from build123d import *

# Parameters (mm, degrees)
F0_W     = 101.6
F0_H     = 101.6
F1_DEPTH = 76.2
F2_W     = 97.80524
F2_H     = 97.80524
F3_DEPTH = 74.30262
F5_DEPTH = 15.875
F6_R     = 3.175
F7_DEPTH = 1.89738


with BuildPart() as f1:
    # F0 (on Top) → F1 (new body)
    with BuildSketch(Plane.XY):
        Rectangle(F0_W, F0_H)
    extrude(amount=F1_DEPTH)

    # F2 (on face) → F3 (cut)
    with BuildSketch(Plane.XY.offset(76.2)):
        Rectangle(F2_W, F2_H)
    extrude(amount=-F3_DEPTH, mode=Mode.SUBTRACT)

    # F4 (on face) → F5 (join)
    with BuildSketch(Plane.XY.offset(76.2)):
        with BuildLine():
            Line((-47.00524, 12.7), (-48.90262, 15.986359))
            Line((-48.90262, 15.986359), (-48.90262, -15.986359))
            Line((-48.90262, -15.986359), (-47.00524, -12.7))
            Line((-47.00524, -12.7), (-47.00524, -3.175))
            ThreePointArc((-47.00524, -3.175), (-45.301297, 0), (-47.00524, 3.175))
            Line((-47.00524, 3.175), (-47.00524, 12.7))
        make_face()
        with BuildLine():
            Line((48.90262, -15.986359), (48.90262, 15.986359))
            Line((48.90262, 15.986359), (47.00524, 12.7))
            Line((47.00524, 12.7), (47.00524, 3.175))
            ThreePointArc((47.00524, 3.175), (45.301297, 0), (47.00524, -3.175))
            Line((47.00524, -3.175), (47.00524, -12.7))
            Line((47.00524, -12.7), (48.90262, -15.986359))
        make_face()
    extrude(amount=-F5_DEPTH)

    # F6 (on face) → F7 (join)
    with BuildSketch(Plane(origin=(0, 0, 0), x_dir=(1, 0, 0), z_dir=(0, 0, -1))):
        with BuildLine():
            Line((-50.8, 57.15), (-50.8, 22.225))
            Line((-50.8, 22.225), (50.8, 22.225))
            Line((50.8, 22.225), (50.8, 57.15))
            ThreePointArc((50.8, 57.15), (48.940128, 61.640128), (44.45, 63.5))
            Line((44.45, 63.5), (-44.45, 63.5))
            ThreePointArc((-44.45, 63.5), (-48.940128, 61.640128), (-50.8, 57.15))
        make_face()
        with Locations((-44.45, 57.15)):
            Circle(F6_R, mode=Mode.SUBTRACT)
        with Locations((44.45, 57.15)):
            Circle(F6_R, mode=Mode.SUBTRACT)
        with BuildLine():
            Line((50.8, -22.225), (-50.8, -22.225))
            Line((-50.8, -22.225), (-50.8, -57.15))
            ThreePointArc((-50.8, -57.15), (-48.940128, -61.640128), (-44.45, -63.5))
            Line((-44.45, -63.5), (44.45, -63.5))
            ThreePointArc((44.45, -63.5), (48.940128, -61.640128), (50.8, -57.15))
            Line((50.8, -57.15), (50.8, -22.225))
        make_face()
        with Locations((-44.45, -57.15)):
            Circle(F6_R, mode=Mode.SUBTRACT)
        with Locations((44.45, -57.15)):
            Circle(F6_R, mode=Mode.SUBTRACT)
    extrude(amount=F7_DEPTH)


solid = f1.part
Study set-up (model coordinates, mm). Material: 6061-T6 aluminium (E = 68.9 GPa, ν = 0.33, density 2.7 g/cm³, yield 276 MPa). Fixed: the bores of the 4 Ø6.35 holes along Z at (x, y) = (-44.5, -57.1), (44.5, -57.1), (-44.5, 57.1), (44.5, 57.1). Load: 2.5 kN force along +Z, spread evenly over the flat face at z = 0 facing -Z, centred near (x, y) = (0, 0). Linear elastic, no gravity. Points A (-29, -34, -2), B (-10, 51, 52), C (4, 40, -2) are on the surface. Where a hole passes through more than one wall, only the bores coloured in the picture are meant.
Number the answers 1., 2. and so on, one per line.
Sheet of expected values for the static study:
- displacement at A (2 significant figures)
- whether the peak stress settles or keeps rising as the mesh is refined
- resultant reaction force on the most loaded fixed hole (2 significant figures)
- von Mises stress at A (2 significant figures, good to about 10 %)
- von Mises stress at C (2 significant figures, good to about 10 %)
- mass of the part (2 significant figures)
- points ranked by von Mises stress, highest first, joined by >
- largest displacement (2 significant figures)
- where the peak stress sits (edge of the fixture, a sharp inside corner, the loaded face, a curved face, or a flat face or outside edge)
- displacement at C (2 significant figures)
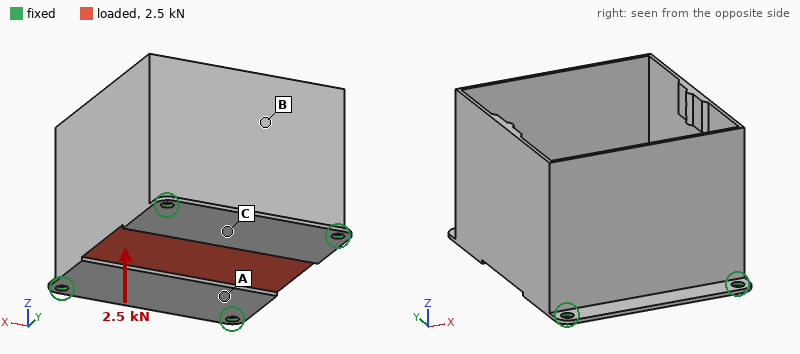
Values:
1. 0.19 mm
2. keeps rising
3. 1.8 kN
4. 91 MPa
5. 38 MPa
6. 250 g
7. A > C > B
8. 0.82 mm
9. edge of the fixture
10. 0.19 mm
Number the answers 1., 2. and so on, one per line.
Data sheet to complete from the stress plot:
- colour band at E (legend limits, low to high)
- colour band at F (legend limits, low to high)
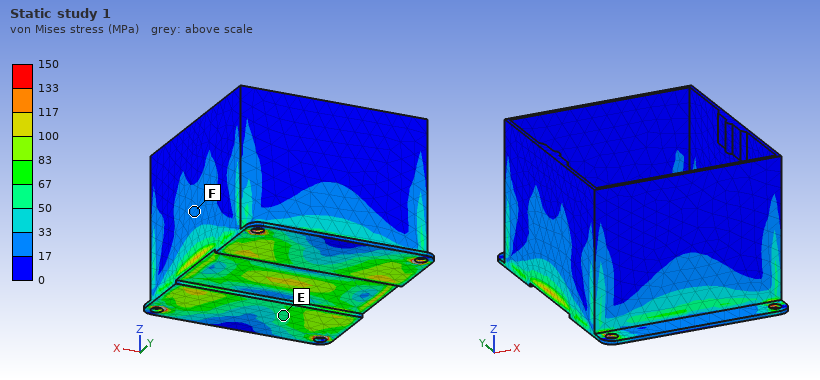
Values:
1. 50 to 67 MPa
2. 17 to 33 MPa
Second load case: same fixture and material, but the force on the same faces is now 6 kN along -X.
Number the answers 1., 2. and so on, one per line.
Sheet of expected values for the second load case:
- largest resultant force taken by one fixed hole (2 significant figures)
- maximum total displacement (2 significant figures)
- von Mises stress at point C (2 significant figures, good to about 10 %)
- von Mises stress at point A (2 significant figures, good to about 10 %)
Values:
1. 1.7 kN
2. 31 µm
3. 15 MPa
4. 15 MPa
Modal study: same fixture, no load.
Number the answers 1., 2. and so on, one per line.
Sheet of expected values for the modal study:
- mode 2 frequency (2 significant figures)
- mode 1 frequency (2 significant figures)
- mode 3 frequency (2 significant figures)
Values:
1. 880 Hz
2. 690 Hz
3. 910 Hz
